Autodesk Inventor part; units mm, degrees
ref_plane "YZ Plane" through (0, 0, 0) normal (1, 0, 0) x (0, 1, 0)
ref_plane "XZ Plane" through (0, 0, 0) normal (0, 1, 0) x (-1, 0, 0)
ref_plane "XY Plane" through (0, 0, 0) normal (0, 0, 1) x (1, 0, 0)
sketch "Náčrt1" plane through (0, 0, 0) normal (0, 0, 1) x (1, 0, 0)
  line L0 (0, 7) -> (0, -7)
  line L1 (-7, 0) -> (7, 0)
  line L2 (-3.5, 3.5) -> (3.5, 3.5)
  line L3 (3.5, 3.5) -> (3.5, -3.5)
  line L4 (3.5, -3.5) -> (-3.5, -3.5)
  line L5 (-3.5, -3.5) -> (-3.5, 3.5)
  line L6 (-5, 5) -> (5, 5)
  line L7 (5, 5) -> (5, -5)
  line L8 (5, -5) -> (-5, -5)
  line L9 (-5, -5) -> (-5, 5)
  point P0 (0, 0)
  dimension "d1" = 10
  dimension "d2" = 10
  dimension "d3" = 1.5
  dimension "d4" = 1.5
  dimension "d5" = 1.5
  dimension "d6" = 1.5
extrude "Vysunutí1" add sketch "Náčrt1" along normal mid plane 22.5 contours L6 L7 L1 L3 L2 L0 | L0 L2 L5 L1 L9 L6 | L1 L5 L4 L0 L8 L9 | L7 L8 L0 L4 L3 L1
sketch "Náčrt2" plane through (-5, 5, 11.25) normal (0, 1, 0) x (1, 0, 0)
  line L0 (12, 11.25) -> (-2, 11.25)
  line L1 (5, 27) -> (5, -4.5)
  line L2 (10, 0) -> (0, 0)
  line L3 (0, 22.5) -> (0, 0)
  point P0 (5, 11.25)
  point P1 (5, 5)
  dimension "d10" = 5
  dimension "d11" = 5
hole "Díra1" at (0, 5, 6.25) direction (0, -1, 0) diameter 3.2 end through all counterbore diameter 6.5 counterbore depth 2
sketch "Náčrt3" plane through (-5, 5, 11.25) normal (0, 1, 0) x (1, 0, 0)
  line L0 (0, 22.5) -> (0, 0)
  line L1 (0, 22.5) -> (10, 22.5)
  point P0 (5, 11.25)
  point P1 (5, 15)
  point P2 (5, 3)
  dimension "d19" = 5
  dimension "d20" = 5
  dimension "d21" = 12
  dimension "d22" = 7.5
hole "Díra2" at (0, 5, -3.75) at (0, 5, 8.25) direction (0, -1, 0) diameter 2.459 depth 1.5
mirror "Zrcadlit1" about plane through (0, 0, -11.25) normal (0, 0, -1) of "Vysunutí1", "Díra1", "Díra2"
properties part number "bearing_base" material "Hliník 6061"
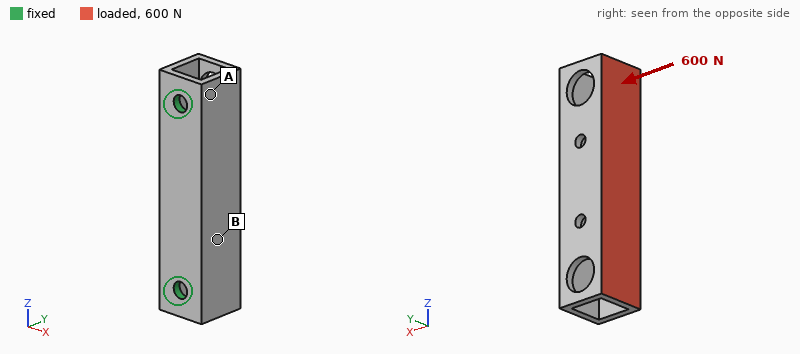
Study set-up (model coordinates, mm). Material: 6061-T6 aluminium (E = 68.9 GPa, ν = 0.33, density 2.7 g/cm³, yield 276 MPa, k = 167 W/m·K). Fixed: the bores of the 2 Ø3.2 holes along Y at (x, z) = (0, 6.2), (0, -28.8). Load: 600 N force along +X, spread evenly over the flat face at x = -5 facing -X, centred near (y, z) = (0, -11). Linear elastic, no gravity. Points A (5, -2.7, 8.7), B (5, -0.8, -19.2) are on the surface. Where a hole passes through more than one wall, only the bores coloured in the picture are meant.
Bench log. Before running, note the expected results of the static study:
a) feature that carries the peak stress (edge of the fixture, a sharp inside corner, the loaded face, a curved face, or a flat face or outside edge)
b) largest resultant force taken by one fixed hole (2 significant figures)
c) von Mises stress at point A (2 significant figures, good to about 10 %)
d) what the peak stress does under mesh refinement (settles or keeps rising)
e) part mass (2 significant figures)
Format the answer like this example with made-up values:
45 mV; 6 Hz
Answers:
edge of the fixture; 300 N; 37 MPa; keeps rising; 5.8 g
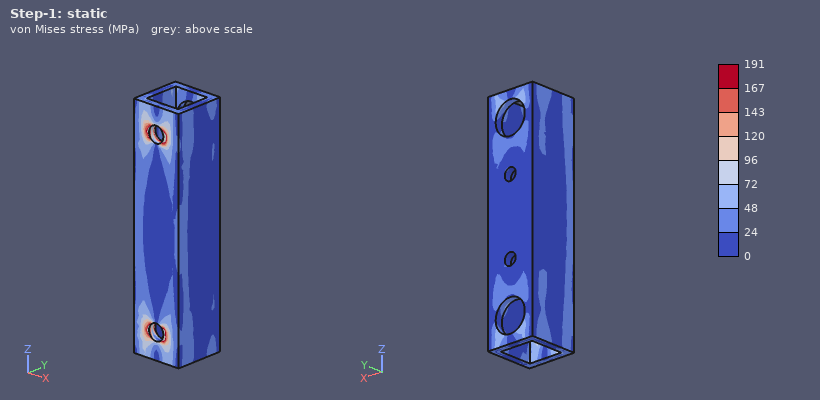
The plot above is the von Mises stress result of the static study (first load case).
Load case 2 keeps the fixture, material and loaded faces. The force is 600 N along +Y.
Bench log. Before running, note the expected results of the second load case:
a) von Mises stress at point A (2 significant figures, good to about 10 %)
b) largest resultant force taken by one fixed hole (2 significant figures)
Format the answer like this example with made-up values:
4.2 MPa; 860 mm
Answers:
31 MPa; 330 N
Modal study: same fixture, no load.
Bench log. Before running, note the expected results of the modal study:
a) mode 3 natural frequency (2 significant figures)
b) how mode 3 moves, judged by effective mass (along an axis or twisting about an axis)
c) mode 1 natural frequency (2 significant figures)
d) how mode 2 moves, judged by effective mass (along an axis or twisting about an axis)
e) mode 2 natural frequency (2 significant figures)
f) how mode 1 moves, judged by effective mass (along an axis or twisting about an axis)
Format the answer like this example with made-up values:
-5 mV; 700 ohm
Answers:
20 kHz; twisting about Y; 6900 Hz; along Y; 16 kHz; along X
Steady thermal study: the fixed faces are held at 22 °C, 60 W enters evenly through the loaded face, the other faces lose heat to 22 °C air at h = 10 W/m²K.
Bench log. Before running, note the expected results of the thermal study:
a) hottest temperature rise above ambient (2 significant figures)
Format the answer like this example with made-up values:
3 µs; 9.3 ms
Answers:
58 K
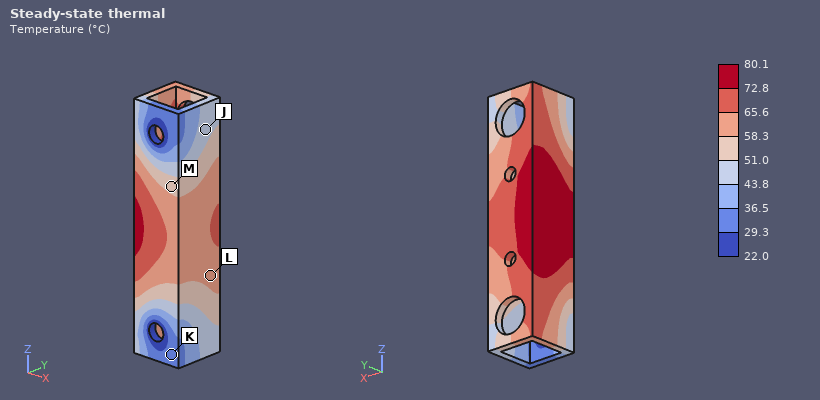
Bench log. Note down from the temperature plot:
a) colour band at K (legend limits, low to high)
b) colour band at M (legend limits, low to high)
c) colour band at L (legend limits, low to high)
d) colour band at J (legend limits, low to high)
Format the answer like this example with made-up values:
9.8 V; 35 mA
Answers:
29.3 to 36.5 °C; 51.0 to 58.3 °C; 58.3 to 65.6 °C; 43.8 to 51.0 °C
